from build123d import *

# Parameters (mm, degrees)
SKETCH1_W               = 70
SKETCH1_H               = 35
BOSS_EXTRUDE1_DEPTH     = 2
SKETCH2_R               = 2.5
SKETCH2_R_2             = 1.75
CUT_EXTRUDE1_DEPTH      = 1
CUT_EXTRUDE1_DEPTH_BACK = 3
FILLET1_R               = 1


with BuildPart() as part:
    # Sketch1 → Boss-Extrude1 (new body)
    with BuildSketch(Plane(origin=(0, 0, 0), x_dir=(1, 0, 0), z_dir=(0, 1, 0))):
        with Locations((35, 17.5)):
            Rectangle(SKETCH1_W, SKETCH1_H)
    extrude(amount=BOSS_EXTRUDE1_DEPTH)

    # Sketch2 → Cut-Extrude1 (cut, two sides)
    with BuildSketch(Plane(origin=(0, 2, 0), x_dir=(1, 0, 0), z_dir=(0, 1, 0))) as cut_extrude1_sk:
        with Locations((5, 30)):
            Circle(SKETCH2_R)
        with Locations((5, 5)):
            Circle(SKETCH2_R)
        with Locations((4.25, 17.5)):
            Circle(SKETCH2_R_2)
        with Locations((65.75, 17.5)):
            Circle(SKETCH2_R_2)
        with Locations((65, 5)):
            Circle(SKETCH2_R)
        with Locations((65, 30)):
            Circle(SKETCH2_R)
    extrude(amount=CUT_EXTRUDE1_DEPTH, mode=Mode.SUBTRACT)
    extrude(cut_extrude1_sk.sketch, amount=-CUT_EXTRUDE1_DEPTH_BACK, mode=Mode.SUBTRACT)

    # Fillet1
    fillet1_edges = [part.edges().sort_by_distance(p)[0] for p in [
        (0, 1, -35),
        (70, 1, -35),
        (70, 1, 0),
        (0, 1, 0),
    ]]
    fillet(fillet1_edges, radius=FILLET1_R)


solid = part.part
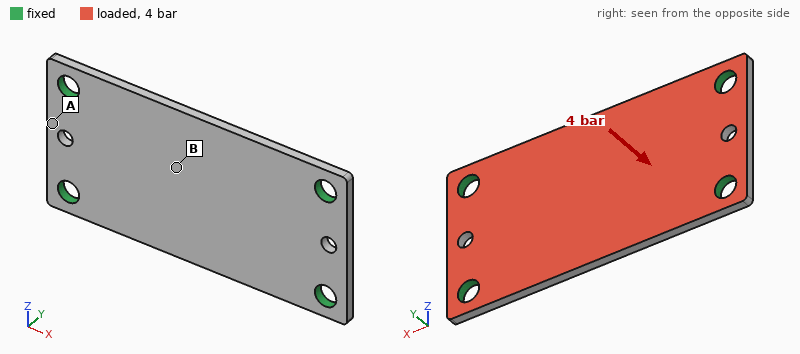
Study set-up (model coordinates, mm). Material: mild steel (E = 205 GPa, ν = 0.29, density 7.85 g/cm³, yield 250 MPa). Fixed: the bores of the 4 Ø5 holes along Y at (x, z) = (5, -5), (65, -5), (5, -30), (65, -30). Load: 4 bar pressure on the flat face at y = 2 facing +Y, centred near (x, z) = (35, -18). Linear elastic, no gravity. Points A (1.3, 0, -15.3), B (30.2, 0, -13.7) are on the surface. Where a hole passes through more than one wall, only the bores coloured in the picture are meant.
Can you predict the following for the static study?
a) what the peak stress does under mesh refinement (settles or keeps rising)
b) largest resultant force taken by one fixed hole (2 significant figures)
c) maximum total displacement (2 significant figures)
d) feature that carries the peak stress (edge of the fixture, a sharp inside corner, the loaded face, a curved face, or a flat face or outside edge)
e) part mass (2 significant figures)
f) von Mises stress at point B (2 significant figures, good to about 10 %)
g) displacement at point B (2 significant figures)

keeps rising
240 N
90 µm
edge of the fixture
37 g
68 MPa
82 µm
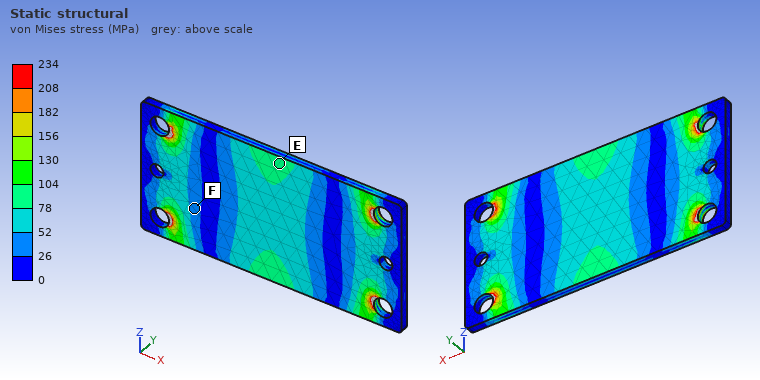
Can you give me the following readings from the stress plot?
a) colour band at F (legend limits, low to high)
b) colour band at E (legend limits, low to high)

26 to 52 MPa
78 to 104 MPa
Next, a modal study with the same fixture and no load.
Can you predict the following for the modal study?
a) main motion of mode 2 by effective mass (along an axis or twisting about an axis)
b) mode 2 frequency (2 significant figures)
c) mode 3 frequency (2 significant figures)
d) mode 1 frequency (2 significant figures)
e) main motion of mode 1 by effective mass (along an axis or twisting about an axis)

twisting about X
4800 Hz
8400 Hz
3100 Hz
along Y
